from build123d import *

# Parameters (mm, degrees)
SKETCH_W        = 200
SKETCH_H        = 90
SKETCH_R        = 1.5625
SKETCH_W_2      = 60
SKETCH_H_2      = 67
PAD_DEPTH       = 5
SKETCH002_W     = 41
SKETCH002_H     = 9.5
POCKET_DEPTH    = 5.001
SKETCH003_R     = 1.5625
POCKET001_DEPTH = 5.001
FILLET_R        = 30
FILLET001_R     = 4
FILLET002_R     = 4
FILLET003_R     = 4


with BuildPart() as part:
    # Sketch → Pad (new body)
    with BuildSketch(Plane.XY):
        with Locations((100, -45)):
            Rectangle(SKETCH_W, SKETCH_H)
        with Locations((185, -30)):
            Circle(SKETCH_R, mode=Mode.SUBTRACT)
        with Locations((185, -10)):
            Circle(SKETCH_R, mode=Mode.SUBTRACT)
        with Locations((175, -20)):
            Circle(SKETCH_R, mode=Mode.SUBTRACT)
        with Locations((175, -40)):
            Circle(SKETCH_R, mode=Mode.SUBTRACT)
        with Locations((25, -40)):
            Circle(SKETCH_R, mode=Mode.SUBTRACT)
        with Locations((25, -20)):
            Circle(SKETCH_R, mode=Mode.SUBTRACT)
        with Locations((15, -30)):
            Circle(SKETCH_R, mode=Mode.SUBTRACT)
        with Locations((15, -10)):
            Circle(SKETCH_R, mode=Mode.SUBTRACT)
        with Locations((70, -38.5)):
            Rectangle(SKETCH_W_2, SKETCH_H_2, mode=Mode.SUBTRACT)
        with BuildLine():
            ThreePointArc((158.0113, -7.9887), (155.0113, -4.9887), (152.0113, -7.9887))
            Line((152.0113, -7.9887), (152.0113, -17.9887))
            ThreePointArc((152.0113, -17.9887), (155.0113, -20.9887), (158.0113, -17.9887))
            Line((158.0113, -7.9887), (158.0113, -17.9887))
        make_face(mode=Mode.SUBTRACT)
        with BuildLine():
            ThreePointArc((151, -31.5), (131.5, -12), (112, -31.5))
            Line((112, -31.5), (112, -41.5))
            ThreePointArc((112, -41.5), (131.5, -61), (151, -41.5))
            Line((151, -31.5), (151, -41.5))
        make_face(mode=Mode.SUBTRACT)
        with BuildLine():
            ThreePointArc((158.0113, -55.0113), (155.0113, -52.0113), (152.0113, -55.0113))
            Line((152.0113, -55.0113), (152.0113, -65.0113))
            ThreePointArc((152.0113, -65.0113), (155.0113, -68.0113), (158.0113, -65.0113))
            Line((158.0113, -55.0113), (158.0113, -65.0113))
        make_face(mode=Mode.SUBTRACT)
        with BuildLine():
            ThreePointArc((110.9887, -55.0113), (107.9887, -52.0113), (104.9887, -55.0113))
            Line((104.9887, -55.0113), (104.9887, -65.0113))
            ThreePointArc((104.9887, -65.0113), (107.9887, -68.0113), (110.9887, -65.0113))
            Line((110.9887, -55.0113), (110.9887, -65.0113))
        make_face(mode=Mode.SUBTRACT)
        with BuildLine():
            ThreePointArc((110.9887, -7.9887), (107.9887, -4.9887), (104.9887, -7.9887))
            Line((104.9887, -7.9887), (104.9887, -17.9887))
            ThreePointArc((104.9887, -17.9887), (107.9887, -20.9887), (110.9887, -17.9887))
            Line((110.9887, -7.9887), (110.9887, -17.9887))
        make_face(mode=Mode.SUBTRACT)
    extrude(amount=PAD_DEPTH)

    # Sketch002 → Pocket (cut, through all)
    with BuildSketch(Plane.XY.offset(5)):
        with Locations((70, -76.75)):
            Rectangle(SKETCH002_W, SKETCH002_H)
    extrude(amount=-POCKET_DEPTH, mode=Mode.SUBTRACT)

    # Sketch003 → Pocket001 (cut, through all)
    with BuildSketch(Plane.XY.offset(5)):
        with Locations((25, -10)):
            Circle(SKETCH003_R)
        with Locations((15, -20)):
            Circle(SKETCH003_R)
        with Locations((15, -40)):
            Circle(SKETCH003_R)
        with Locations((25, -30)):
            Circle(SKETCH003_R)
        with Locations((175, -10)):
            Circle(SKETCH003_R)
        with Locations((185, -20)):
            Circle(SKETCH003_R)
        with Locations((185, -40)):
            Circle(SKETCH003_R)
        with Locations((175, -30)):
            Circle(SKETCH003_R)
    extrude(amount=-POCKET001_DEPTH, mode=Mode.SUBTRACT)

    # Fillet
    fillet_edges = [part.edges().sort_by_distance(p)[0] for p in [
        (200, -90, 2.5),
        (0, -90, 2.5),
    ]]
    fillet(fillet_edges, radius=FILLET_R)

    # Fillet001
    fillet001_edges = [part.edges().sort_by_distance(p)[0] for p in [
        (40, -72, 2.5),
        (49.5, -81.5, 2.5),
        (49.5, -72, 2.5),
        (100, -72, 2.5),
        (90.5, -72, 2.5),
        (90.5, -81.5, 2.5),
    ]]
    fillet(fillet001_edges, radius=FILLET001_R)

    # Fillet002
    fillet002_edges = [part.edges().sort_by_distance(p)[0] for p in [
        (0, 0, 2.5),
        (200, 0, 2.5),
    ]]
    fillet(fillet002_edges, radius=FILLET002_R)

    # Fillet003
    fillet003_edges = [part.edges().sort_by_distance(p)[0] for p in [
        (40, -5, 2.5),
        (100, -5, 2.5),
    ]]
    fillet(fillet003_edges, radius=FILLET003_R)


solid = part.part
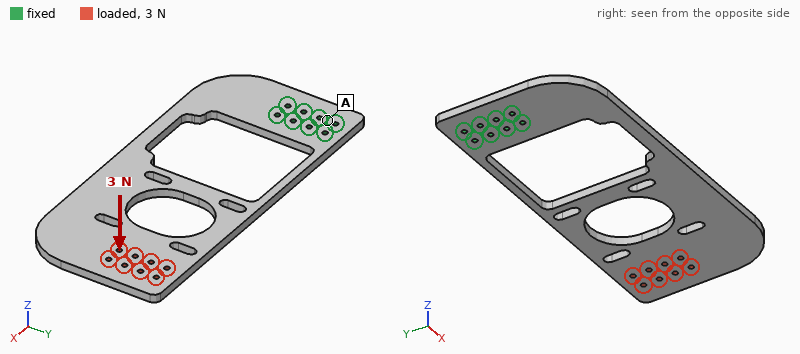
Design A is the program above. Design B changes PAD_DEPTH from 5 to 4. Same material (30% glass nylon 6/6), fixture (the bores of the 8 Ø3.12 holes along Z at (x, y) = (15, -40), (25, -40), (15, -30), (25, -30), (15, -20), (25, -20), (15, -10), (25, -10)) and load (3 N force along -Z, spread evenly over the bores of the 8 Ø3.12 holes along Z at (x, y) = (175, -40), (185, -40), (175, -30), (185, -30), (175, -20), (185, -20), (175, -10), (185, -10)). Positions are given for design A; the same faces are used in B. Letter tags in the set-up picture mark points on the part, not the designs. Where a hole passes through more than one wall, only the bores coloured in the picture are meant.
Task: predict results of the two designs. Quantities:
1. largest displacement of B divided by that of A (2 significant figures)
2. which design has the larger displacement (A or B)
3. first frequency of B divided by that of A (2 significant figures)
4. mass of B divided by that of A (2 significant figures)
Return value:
1.9
B
0.80
0.80
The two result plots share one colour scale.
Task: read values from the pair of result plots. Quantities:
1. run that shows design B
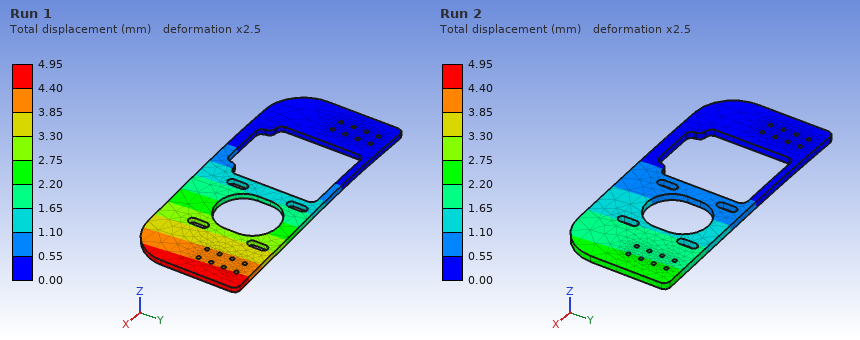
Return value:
Run 1
